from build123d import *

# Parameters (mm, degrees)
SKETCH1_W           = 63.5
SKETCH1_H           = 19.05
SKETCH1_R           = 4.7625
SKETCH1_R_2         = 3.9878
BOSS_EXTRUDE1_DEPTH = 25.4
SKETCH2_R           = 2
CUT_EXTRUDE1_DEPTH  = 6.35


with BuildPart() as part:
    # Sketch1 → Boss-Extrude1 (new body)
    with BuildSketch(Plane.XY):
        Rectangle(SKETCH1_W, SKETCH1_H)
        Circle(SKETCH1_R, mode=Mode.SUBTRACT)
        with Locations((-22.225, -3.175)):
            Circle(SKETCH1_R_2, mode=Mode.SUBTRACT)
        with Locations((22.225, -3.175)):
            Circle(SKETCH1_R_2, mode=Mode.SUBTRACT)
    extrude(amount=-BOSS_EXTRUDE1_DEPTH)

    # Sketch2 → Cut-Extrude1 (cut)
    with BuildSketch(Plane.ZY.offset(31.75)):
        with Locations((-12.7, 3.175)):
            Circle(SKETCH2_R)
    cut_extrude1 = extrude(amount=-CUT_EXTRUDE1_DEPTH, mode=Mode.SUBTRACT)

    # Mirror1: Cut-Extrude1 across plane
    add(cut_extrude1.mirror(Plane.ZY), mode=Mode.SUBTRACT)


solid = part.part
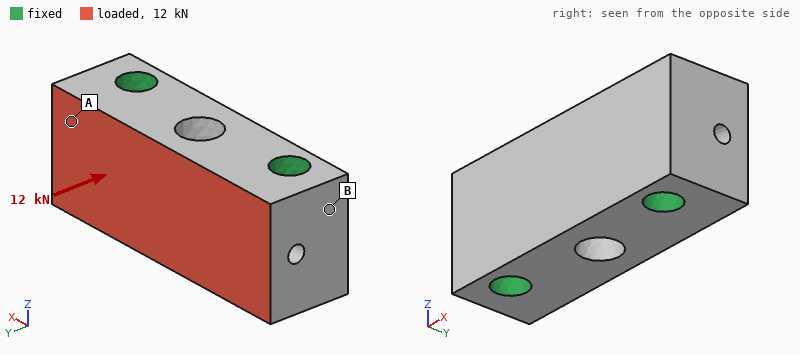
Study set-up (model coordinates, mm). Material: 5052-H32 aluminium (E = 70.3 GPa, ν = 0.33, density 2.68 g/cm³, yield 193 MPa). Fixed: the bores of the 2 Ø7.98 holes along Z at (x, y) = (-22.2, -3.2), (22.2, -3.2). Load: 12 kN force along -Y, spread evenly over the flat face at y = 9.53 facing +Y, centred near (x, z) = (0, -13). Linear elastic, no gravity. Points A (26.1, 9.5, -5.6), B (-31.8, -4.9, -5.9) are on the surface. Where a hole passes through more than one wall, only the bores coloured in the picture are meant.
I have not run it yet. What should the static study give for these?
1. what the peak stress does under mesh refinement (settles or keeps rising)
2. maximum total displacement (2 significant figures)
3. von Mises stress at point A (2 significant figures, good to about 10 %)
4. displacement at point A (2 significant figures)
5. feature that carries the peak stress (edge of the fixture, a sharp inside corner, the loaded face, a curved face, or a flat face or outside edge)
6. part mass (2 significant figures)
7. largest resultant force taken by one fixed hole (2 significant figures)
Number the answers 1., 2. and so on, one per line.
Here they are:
1. keeps rising
2. 7.2 µm
3. 11 MPa
4. 1.3 µm
5. edge of the fixture
6. 70 g
7. 6.1 kN
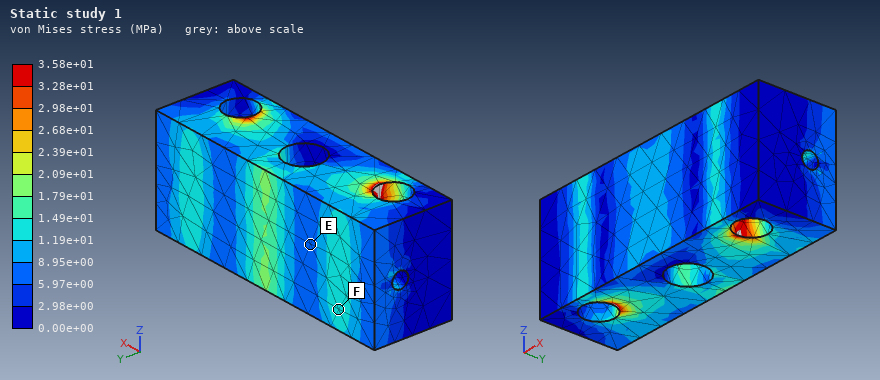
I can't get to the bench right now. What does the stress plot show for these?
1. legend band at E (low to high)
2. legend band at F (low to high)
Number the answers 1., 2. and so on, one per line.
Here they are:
1. 5.97e+00 to 8.95e+00 MPa
2. 1.19e+01 to 1.49e+01 MPa
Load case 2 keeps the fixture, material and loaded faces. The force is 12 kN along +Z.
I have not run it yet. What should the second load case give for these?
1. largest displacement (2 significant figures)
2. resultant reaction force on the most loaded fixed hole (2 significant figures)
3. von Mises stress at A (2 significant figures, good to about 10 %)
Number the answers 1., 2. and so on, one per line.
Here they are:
1. 16 µm
2. 6.0 kN
3. 16 MPa
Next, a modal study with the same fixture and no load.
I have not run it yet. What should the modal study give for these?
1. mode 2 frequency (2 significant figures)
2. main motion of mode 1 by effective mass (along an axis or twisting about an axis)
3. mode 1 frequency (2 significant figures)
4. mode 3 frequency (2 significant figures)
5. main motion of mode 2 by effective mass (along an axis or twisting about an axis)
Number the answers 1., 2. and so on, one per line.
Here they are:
1. 33 kHz
2. along Y
3. 30 kHz
4. 37 kHz
5. along Z
